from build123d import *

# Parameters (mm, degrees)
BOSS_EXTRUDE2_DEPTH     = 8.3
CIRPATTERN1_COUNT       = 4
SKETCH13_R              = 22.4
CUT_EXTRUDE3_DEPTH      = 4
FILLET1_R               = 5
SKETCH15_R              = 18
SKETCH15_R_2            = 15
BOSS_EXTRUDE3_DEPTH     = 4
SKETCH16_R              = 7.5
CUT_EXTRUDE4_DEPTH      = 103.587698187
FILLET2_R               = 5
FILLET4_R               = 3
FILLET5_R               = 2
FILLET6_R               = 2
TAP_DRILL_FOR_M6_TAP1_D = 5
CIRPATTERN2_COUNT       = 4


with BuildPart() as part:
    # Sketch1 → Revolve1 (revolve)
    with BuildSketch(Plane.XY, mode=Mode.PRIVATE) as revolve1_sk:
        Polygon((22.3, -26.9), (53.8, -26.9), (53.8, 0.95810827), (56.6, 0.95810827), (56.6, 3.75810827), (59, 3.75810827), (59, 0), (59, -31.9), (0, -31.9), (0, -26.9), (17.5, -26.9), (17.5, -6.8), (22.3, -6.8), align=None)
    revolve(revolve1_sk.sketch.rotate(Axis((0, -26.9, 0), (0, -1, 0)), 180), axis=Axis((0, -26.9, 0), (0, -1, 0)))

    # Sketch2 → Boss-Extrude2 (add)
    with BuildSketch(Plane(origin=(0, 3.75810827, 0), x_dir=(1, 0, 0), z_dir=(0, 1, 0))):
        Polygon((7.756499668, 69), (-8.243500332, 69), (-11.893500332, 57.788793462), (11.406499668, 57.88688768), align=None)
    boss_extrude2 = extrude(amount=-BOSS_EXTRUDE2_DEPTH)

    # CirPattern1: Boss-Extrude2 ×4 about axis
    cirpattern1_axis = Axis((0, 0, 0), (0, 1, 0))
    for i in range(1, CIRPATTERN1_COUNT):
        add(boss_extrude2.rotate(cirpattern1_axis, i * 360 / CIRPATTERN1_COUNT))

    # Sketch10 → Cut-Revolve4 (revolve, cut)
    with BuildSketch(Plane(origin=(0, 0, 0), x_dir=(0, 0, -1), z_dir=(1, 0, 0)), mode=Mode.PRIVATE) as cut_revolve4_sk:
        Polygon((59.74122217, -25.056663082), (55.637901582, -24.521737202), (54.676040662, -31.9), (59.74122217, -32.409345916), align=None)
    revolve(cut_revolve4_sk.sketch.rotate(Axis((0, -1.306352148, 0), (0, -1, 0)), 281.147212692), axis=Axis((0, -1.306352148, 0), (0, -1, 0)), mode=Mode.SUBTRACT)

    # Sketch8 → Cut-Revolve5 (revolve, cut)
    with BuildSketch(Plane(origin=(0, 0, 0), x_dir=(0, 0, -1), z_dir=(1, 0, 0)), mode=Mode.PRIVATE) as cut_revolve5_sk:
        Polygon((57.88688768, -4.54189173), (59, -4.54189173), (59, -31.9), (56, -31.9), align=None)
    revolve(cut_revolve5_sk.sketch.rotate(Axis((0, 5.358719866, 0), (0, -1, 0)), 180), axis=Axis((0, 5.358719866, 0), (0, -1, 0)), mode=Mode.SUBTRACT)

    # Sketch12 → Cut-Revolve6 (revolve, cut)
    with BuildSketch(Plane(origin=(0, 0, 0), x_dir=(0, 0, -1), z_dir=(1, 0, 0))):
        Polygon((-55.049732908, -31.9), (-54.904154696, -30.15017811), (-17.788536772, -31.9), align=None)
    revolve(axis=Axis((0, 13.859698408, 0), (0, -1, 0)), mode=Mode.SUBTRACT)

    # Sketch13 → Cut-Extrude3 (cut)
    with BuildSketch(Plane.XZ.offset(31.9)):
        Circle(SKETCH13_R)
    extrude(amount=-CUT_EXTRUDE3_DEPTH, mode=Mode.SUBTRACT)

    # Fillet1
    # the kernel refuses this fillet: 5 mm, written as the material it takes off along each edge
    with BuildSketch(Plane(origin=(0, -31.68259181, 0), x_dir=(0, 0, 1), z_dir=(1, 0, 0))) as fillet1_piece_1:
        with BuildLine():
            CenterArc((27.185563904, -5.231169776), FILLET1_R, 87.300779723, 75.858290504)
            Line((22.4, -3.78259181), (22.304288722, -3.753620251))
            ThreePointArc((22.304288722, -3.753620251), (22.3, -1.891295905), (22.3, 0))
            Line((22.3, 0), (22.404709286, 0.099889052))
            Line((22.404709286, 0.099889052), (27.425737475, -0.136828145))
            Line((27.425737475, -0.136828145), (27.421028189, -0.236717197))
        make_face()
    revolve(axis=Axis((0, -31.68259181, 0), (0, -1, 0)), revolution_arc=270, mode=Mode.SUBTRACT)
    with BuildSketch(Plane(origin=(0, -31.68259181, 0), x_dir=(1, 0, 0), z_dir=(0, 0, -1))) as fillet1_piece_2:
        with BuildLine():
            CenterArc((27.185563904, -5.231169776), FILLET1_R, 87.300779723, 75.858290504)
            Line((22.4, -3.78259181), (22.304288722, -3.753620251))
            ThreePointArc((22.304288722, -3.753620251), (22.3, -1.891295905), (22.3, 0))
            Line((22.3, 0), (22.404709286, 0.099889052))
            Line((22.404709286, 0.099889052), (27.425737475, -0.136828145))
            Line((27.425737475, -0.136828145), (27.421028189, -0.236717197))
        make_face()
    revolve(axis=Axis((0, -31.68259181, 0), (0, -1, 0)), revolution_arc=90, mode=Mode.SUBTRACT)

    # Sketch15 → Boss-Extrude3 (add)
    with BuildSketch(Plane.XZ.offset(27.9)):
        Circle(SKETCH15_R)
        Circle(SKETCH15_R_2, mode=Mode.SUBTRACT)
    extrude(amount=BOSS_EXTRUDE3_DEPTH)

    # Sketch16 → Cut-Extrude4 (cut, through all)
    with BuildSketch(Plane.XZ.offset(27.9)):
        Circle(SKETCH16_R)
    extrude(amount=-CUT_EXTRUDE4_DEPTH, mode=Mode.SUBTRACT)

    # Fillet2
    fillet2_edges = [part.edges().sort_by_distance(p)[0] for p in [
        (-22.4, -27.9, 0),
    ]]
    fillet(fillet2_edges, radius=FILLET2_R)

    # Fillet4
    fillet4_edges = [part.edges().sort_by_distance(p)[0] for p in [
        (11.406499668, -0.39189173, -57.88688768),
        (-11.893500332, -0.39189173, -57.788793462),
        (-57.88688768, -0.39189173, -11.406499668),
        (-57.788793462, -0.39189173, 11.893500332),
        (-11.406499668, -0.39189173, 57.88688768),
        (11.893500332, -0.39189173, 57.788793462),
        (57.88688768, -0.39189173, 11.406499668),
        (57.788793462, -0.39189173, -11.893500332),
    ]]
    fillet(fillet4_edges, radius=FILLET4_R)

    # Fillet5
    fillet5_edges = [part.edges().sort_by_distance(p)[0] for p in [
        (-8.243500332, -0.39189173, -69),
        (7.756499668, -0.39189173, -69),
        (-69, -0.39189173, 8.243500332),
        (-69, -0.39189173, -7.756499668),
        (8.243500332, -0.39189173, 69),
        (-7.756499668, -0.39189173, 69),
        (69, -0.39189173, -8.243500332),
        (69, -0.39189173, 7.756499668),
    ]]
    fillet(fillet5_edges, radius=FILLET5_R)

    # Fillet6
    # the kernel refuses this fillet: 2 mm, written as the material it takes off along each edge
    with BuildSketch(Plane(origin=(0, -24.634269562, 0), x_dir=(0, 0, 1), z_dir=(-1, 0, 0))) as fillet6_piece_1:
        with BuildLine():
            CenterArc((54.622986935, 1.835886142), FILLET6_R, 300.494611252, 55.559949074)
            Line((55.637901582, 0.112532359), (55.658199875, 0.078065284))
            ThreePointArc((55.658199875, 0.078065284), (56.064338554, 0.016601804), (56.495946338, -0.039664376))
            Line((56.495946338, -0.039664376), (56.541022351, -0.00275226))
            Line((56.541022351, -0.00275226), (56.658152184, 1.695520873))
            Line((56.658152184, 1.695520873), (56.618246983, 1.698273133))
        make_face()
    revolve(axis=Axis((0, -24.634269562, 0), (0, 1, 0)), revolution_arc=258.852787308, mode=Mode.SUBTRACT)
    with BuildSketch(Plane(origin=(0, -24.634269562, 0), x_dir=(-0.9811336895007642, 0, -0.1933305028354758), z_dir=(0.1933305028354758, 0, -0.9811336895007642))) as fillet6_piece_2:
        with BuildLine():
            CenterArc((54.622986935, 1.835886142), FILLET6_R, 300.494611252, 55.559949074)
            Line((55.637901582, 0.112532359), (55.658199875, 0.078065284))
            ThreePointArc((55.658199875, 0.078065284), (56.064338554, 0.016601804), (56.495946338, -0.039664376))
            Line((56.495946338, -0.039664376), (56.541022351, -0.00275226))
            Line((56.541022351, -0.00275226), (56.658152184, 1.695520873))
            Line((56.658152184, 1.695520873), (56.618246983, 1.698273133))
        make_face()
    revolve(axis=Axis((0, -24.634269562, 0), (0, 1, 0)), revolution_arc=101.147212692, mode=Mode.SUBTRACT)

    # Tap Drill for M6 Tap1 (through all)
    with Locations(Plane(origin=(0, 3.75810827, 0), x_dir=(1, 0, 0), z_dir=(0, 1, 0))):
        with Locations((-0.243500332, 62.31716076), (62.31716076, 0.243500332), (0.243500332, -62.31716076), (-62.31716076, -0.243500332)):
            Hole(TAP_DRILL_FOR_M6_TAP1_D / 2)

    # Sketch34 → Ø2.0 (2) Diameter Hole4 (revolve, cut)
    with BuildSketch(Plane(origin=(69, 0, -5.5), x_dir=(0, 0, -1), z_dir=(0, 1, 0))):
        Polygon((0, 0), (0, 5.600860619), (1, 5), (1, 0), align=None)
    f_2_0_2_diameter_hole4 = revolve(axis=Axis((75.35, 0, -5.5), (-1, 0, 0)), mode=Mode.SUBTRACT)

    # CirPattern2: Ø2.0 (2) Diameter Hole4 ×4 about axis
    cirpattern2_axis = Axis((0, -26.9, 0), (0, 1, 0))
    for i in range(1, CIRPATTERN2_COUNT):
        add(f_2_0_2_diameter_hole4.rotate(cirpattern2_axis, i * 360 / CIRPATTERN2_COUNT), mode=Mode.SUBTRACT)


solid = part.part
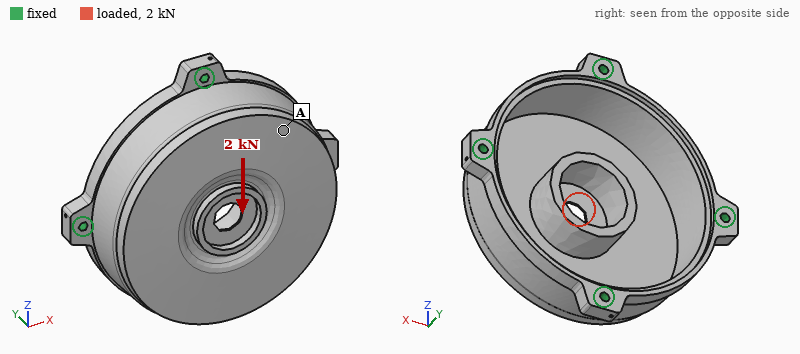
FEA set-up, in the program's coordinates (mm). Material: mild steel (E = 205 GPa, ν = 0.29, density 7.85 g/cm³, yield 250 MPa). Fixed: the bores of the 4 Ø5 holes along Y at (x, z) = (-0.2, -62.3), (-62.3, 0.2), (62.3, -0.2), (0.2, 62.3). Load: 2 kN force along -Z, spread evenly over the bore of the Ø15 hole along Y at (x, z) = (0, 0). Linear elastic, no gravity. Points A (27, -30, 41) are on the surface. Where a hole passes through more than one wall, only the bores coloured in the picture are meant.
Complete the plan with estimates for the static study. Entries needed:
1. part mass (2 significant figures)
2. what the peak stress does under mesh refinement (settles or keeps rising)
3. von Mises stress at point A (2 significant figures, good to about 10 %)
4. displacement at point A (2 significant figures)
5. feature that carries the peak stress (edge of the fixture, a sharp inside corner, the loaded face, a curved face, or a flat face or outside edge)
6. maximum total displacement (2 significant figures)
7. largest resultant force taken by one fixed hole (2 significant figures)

700 g
keeps rising
6.1 MPa
4.0 µm
a sharp inside corner
7.1 µm
700 N
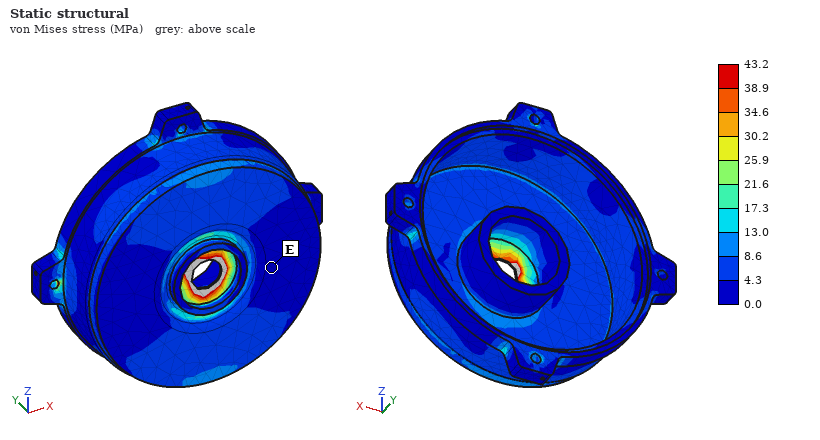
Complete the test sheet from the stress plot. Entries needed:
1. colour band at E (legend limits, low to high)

0.0 to 4.3 MPa
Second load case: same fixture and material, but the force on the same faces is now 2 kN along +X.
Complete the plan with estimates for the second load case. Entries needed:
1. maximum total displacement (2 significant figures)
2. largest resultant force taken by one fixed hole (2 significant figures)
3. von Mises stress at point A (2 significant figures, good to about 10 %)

7.1 µm
700 N
4.0 MPa
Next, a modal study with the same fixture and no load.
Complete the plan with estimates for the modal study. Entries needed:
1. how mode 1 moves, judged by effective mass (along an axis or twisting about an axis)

along Y
